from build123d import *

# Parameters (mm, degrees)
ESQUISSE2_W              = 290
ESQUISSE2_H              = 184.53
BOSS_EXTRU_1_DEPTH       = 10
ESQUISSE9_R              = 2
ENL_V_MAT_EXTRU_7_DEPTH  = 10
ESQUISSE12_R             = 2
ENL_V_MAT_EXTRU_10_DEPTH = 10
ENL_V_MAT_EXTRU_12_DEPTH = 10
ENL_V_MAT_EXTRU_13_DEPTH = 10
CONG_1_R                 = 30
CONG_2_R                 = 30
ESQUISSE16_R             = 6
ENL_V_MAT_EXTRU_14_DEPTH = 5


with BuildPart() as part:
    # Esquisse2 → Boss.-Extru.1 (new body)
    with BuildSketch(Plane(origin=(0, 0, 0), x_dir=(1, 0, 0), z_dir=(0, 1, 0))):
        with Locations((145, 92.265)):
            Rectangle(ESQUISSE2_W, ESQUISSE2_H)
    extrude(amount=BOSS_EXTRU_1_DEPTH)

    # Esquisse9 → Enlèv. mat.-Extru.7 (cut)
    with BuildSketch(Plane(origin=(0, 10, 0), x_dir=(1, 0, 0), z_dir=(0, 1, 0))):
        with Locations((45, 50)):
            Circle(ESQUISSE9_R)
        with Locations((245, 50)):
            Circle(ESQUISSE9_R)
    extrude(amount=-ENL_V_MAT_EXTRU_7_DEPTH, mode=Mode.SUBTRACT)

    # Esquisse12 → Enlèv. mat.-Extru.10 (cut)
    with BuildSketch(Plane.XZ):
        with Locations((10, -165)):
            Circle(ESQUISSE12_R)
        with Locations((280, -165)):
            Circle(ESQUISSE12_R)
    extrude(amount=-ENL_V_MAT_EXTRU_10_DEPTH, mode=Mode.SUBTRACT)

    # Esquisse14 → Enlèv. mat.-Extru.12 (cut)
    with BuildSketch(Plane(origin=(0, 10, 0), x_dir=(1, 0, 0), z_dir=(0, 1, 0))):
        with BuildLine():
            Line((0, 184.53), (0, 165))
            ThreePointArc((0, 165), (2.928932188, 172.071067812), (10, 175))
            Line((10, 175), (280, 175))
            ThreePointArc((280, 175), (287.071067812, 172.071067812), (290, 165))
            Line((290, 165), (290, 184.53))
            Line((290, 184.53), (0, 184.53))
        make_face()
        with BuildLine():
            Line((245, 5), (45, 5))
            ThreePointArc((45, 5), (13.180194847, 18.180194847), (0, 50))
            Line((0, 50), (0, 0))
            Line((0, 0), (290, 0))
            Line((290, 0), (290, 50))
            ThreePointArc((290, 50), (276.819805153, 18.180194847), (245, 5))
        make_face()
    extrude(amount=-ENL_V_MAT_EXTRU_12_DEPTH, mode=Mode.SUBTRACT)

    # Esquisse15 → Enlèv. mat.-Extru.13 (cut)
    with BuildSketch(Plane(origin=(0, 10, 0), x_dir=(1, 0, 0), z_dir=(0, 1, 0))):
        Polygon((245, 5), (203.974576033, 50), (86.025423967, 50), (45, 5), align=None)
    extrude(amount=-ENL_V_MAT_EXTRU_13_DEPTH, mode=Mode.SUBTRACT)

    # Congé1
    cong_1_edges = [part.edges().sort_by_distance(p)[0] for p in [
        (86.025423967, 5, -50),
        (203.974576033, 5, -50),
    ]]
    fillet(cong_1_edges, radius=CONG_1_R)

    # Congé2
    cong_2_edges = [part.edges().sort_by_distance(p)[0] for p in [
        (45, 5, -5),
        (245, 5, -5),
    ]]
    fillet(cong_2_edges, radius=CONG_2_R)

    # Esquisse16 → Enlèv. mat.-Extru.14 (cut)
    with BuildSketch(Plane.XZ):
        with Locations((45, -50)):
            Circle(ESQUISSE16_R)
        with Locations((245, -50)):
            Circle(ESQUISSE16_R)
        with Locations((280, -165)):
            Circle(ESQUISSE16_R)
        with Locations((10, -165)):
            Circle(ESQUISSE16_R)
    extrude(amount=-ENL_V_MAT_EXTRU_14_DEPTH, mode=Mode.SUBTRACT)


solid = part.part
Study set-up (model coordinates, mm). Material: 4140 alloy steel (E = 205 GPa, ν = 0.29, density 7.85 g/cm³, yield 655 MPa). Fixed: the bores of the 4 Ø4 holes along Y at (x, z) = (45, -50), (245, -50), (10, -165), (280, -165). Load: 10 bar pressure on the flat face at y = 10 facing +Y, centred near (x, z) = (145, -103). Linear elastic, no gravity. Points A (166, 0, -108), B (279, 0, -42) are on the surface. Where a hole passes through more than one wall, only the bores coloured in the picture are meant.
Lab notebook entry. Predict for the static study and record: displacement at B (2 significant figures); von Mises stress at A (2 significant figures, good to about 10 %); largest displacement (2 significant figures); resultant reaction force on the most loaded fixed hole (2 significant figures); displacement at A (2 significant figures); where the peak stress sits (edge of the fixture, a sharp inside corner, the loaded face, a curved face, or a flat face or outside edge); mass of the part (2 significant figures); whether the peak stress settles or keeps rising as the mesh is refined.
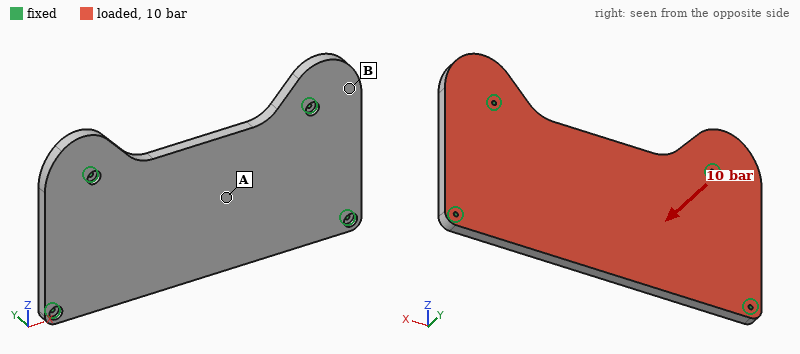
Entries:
0.25 mm
200 MPa
1.5 mm
21 kN
1.00 mm
edge of the fixture
3.2 kg
keeps rising
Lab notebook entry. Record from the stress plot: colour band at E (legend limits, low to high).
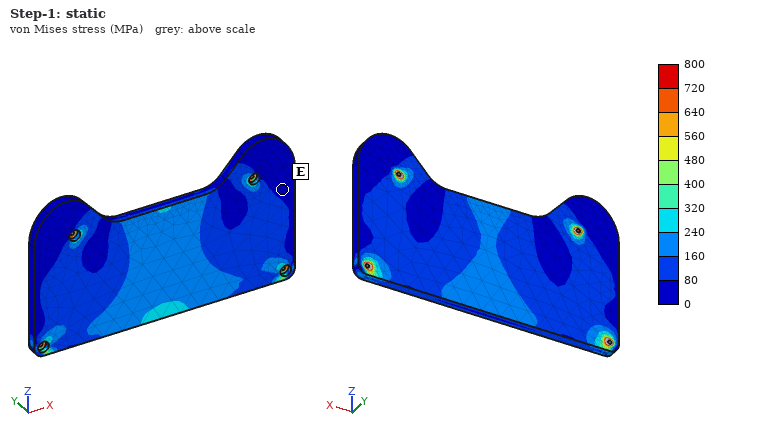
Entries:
0 to 80 MPa
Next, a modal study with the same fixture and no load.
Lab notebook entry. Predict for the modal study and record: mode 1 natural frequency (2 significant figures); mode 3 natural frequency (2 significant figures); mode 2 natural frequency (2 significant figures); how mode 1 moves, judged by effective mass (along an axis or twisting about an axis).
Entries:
580 Hz
1600 Hz
1400 Hz
along Y
